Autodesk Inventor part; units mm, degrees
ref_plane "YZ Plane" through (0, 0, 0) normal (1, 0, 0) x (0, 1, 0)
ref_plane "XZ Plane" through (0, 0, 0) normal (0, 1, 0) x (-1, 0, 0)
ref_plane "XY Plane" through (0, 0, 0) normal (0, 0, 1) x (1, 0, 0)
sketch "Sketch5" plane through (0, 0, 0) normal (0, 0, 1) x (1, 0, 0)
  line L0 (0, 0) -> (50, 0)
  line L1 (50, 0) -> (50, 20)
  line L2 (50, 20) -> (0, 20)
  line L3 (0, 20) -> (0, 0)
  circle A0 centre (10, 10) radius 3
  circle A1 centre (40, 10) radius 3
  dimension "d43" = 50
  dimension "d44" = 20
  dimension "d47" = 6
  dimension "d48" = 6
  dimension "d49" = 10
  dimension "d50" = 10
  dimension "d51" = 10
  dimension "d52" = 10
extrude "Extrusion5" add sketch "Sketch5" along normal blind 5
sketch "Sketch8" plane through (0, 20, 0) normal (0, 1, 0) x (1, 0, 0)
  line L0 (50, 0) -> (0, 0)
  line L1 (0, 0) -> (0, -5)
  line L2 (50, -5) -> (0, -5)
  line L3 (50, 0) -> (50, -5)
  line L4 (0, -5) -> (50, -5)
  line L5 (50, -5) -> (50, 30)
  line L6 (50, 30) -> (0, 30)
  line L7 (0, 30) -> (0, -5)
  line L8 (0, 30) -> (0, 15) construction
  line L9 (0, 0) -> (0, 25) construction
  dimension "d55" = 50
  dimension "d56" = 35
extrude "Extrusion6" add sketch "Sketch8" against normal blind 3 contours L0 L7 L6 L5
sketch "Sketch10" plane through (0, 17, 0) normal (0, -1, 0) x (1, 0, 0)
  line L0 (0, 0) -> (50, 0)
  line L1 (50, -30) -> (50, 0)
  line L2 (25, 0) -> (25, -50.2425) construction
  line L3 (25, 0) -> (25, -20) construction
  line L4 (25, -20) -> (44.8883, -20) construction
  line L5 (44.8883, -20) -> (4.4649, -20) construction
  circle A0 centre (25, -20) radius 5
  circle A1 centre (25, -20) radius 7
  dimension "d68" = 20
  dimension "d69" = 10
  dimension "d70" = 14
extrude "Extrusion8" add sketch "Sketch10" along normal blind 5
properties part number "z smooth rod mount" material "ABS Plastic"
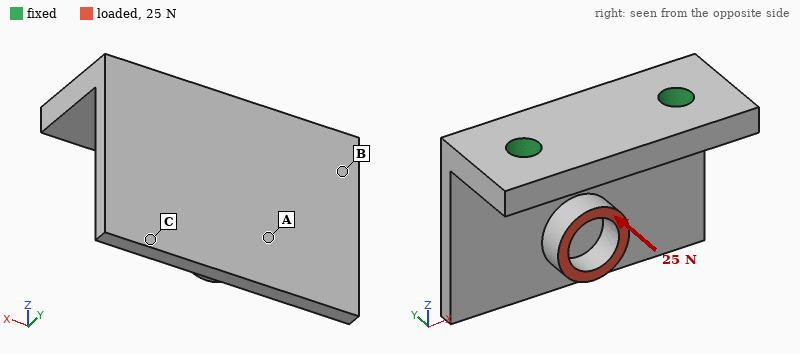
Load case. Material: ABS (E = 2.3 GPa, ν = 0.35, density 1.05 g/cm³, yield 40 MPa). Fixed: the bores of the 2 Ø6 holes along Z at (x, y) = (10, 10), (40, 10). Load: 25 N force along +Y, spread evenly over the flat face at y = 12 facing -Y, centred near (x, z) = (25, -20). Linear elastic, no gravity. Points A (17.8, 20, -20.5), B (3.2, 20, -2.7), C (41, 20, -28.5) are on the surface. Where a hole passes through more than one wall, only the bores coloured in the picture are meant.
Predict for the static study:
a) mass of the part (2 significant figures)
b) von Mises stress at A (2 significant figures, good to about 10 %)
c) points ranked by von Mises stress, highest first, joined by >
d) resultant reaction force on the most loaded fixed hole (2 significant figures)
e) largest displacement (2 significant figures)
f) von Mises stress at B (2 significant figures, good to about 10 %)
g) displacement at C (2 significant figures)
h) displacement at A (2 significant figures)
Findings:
10 g
1.6 MPa
B > A > C
13 N
0.65 mm
4.9 MPa
0.56 mm
0.40 mm
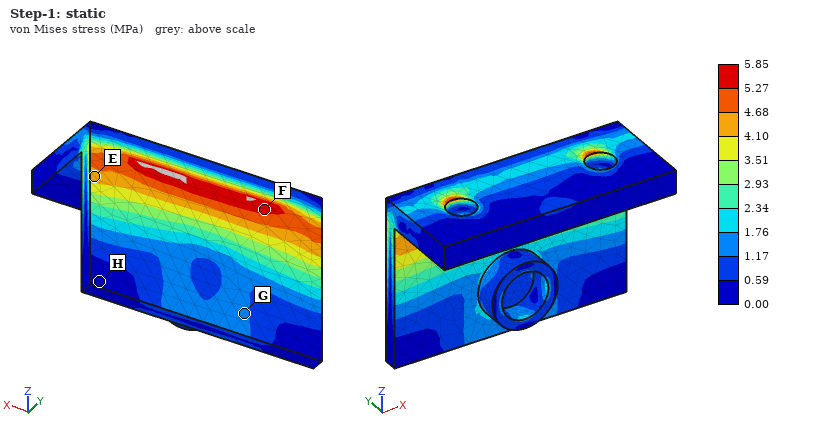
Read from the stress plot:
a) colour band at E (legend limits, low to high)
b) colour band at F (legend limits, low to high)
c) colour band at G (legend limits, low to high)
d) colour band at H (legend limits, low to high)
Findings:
4.10 to 4.68 MPa
5.27 to 5.85 MPa
1.17 to 1.76 MPa
0.00 to 0.59 MPa
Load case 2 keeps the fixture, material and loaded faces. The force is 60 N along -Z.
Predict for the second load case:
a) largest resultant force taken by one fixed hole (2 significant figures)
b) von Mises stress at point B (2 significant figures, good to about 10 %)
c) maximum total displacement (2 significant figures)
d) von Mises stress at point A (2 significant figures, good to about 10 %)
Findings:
31 N
4.2 MPa
0.66 mm
2.1 MPa
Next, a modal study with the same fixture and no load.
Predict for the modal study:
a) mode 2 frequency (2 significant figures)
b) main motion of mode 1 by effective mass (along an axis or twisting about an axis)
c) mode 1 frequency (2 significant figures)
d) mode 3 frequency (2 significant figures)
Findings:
1300 Hz
along Y
650 Hz
2800 Hz
